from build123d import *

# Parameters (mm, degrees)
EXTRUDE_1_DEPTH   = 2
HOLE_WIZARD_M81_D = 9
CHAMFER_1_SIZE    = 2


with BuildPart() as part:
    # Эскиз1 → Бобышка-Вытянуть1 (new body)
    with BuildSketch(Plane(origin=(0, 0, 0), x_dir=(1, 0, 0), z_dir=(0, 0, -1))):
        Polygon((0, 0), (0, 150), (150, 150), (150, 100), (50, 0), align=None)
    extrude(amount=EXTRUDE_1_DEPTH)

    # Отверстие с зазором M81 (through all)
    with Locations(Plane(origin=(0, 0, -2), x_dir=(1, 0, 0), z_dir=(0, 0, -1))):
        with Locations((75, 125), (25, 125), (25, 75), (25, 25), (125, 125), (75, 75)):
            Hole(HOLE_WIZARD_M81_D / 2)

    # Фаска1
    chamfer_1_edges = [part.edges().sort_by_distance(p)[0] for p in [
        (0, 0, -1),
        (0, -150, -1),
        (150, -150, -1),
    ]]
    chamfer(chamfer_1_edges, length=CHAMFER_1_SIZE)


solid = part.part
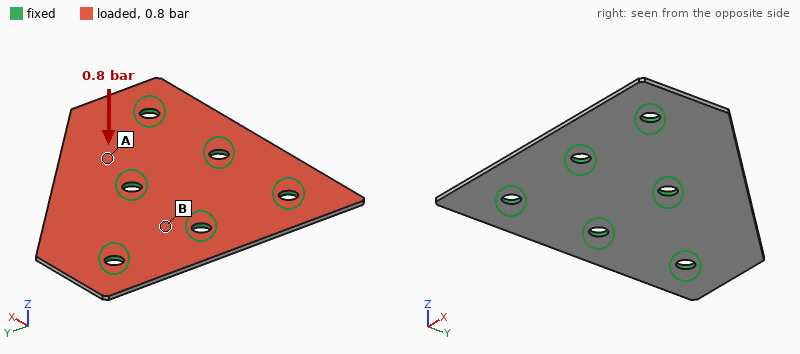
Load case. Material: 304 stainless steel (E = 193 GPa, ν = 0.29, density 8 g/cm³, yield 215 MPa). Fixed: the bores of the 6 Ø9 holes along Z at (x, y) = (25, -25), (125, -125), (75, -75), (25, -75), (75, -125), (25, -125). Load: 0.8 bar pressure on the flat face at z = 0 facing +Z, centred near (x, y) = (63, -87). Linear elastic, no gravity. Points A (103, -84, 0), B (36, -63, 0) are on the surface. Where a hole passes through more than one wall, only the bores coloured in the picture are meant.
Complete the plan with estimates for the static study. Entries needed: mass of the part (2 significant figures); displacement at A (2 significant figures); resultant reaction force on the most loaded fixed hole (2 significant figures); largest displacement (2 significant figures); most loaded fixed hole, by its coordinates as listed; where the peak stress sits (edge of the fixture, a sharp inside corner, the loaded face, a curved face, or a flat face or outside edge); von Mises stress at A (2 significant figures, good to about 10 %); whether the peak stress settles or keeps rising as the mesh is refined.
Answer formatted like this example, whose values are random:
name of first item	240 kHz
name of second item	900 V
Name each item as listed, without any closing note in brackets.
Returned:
mass of the part	270 g
displacement at A	0.059 mm
resultant reaction force on the most loaded fixed hole	320 N
largest displacement	0.14 mm
most loaded fixed hole, by its coordinates as listed	(75, -75)
where the peak stress sits	edge of the fixture
von Mises stress at A	26 MPa
whether the peak stress settles or keeps rising as the mesh is refined	keeps rising
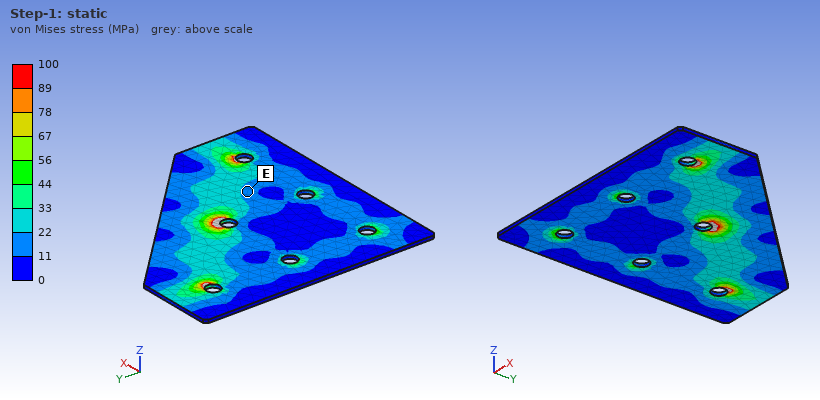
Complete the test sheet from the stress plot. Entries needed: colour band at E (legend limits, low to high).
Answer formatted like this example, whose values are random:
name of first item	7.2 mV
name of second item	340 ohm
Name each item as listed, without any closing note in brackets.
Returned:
colour band at E	11 to 22 MPa
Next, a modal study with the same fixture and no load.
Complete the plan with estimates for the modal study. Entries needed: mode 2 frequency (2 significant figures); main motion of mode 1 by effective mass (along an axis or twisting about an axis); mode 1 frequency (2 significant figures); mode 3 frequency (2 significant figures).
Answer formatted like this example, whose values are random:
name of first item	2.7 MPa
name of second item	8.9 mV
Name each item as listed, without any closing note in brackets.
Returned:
mode 2 frequency	1400 Hz
main motion of mode 1 by effective mass	along Z
mode 1 frequency	1200 Hz
mode 3 frequency	2300 Hz
